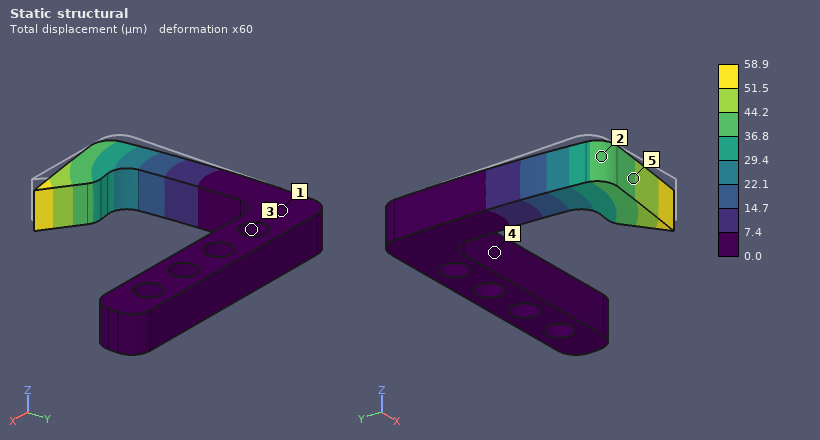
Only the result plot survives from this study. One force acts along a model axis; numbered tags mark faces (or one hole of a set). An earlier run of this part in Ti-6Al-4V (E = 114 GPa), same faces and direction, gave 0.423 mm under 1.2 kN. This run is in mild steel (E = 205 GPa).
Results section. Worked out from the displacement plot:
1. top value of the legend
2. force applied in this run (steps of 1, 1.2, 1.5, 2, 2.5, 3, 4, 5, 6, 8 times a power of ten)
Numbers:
58.9 µm
300 N
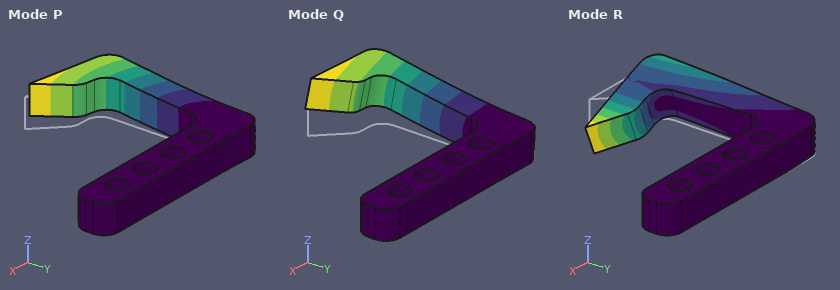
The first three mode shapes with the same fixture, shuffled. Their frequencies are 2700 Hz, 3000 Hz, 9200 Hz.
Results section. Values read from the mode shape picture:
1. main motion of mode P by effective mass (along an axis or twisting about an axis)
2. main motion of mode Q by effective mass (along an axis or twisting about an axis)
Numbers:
along X
along Z
